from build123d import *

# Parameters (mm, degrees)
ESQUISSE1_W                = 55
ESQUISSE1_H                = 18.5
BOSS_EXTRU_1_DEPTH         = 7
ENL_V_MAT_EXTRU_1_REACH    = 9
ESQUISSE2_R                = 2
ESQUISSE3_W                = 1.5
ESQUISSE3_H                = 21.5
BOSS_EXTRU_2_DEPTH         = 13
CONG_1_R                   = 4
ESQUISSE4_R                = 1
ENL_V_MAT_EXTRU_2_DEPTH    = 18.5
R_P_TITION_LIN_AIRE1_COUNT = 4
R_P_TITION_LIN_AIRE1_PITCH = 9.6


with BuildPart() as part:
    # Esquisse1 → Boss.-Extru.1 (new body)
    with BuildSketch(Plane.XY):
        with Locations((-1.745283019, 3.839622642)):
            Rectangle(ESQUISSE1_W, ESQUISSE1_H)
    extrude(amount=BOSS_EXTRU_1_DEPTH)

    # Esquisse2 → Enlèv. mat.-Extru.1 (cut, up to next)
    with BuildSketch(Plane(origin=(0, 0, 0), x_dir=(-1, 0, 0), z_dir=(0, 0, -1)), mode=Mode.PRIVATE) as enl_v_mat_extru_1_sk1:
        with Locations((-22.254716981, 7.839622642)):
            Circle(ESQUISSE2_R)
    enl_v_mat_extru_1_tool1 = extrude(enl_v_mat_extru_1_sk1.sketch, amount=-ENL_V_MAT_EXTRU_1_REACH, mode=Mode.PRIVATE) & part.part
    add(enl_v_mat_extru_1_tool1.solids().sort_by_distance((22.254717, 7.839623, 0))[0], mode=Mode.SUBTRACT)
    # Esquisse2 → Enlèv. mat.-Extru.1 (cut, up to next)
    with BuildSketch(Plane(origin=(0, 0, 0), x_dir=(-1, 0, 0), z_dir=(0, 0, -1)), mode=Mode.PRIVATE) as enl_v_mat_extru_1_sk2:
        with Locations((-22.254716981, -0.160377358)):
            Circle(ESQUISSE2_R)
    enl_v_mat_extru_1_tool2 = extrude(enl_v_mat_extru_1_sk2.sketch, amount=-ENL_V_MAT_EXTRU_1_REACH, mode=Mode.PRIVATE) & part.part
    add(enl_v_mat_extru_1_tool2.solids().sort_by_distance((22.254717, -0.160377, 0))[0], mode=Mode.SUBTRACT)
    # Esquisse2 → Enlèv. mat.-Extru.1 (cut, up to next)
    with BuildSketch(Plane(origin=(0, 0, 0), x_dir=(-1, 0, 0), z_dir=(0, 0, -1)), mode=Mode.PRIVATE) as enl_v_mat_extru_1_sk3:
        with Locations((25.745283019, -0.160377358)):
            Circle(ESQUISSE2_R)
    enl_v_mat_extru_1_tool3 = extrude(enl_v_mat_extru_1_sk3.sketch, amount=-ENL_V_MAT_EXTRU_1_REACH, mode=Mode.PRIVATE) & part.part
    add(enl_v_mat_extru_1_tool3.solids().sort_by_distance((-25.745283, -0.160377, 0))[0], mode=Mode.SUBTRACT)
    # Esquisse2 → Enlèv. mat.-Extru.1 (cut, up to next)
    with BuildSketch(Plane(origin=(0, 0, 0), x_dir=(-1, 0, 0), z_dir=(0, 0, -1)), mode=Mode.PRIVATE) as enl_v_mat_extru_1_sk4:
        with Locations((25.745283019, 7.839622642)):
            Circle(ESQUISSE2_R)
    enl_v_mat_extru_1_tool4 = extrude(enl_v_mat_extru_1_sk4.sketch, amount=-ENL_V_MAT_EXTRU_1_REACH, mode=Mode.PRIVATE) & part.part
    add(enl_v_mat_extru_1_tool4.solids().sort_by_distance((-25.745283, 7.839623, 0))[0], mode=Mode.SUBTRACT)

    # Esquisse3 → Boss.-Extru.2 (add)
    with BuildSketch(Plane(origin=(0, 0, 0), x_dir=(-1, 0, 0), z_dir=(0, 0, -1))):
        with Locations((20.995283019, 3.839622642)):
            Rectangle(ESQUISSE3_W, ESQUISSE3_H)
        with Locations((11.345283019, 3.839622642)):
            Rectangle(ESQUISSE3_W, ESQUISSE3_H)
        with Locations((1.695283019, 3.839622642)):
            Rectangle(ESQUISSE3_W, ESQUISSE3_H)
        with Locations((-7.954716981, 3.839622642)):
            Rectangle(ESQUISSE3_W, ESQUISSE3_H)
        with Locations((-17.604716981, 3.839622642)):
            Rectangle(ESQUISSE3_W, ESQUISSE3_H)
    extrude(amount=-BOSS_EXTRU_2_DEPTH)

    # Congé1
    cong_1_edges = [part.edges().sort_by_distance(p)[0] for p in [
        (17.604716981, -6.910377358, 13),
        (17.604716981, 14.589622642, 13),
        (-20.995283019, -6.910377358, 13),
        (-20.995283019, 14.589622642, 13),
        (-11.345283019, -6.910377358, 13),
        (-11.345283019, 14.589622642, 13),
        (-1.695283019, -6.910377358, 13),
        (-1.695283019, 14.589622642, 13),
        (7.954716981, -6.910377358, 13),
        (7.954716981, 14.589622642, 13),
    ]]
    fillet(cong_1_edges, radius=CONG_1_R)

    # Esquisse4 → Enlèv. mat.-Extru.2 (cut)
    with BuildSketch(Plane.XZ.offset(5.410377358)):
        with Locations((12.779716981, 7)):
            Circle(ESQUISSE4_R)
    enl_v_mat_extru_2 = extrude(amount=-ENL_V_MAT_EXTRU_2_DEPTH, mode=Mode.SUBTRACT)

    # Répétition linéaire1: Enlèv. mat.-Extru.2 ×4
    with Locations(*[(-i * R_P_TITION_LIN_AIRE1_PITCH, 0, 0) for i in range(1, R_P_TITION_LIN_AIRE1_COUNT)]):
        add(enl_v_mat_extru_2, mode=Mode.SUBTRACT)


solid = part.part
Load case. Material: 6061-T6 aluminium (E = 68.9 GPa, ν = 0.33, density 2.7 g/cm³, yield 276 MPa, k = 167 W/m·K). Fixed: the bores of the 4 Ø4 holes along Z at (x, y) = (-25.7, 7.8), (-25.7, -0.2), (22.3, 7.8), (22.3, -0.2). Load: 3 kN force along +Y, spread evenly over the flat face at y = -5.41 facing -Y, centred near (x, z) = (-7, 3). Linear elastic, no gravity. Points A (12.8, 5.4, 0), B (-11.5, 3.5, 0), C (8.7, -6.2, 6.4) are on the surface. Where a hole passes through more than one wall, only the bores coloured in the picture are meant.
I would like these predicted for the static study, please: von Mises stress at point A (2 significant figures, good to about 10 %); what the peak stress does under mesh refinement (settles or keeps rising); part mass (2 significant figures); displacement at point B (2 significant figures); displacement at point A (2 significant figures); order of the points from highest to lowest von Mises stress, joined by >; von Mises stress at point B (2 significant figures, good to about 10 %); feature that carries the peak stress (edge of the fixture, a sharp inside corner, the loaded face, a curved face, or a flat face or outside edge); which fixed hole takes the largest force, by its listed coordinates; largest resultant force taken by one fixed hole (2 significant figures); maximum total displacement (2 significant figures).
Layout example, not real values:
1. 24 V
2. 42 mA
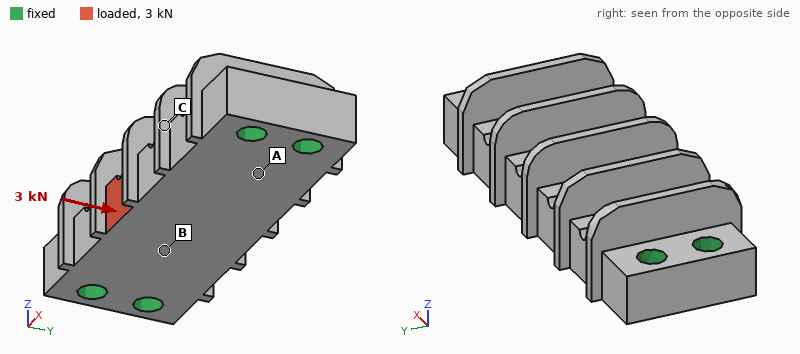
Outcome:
1. 25 MPa
2. keeps rising
3. 21 g
4. 14 µm
5. 5.7 µm
6. B > A > C
7. 38 MPa
8. a sharp inside corner
9. (-25.7, 7.8)
10. 1.7 kN
11. 22 µm
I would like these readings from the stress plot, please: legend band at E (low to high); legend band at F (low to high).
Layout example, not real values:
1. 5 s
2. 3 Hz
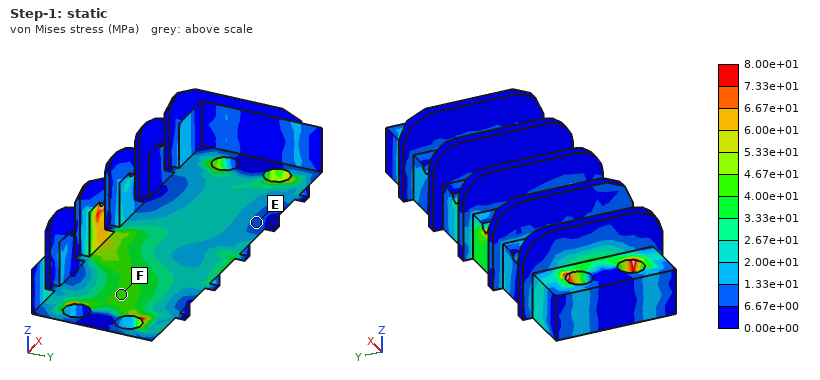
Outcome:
1. 6.67e+00 to 1.33e+01 MPa
2. 4.00e+01 to 4.67e+01 MPa
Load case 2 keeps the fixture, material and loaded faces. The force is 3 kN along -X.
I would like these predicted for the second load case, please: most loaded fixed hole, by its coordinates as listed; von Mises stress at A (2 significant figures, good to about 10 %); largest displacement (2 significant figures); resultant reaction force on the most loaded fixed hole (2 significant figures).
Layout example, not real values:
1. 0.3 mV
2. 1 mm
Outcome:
1. (-25.7, -0.2)
2. 15 MPa
3. 12 µm
4. 1.2 kN
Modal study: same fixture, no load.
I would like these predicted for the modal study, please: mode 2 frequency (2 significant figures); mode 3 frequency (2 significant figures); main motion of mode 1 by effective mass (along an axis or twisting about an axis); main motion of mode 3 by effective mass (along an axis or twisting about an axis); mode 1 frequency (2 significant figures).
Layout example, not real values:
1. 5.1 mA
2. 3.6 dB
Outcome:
1. 19 kHz
2. 23 kHz
3. along Z
4. along Y
5. 14 kHz
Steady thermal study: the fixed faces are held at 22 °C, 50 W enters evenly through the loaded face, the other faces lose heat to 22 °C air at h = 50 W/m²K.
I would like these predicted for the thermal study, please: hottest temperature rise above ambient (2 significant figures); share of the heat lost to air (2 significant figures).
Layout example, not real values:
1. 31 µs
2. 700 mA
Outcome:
1. 43 K
2. 4.7 %
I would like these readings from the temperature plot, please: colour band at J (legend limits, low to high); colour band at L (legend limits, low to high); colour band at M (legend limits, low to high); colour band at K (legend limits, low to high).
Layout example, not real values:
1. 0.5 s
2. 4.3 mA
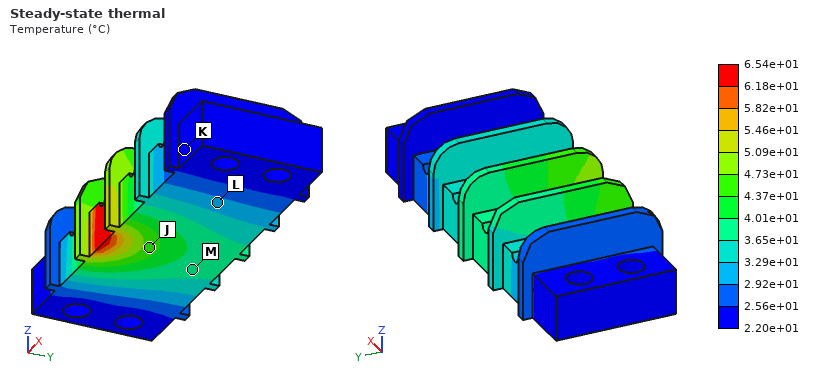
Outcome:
1. 4.37e+01 to 4.73e+01 °C
2. 2.92e+01 to 3.29e+01 °C
3. 3.65e+01 to 4.01e+01 °C
4. 2.20e+01 to 2.56e+01 °C
